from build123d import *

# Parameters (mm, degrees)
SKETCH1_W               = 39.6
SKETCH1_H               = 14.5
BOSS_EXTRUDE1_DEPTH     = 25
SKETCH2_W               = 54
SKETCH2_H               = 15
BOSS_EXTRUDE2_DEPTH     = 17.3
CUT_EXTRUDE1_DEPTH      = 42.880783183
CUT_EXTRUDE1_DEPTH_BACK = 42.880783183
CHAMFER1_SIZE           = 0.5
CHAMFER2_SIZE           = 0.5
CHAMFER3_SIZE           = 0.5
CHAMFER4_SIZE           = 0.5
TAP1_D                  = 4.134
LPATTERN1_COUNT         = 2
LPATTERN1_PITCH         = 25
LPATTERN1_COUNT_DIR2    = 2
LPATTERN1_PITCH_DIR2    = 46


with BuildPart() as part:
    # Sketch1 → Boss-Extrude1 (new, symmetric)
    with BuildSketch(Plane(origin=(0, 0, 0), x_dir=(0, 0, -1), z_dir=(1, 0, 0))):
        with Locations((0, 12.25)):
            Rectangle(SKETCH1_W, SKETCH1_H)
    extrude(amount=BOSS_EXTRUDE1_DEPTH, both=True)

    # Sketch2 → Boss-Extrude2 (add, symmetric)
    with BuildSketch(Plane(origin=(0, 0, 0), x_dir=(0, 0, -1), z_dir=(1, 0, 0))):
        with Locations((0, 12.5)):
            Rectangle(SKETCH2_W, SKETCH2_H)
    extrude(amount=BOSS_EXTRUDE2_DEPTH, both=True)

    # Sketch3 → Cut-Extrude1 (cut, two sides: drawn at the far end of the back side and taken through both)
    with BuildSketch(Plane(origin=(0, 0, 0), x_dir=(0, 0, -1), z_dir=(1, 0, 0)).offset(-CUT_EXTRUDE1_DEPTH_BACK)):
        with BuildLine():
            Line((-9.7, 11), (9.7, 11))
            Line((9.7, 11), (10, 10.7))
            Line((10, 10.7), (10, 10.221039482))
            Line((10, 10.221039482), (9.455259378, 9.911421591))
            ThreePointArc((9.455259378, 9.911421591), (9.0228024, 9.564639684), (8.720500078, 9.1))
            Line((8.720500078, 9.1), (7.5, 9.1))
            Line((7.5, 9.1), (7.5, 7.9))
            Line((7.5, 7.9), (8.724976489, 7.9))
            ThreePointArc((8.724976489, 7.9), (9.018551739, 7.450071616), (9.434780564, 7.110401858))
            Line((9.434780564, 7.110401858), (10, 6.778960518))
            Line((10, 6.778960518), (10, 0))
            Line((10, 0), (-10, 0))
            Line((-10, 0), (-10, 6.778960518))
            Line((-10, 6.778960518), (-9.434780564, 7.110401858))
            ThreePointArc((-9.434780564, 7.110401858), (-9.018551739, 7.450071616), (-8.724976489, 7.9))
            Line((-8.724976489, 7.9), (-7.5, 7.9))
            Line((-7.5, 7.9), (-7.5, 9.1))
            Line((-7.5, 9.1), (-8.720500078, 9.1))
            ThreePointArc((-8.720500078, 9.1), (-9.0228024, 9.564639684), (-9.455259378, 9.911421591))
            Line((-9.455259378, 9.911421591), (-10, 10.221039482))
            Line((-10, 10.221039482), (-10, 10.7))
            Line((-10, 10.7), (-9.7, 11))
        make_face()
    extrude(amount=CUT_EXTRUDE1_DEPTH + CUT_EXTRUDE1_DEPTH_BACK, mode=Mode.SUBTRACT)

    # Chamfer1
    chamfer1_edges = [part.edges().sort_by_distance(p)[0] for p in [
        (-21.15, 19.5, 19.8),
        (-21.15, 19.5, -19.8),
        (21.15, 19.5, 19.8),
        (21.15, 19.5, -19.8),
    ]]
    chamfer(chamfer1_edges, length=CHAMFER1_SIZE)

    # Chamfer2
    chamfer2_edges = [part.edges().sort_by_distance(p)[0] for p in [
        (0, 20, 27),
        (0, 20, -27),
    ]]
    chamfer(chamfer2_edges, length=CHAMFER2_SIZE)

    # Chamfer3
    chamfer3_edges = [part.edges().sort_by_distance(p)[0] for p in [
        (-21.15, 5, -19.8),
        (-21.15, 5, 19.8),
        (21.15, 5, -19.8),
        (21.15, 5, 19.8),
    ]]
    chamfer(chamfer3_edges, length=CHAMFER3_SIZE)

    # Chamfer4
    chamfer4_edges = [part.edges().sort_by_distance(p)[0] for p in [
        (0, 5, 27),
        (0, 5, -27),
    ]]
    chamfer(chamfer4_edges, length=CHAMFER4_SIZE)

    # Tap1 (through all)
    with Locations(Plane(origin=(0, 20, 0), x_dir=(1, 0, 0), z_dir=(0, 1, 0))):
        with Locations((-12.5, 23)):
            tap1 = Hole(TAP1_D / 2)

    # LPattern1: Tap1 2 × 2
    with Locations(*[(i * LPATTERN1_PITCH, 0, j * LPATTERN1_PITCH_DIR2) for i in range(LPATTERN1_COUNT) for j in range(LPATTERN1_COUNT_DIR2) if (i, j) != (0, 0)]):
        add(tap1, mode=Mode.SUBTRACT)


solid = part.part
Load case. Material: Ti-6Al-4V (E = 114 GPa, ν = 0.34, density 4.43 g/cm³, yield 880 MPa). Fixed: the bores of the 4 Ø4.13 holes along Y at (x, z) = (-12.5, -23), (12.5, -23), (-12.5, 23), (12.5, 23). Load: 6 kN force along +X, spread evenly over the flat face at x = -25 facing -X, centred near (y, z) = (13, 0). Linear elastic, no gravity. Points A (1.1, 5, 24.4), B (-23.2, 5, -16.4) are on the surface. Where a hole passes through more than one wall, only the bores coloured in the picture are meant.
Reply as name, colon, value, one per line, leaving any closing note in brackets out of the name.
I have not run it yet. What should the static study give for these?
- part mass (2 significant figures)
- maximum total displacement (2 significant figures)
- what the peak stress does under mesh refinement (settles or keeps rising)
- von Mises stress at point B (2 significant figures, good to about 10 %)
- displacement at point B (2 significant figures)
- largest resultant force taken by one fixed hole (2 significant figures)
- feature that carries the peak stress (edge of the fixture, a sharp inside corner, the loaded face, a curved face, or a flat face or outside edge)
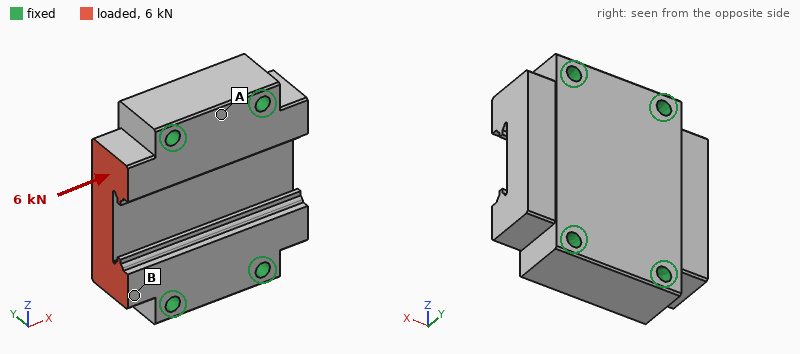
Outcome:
part mass: 140 g
maximum total displacement: 4.0 µm
what the peak stress does under mesh refinement: keeps rising
von Mises stress at point B: 13 MPa
displacement at point B: 2.8 µm
largest resultant force taken by one fixed hole: 1.9 kN
feature that carries the peak stress: edge of the fixture
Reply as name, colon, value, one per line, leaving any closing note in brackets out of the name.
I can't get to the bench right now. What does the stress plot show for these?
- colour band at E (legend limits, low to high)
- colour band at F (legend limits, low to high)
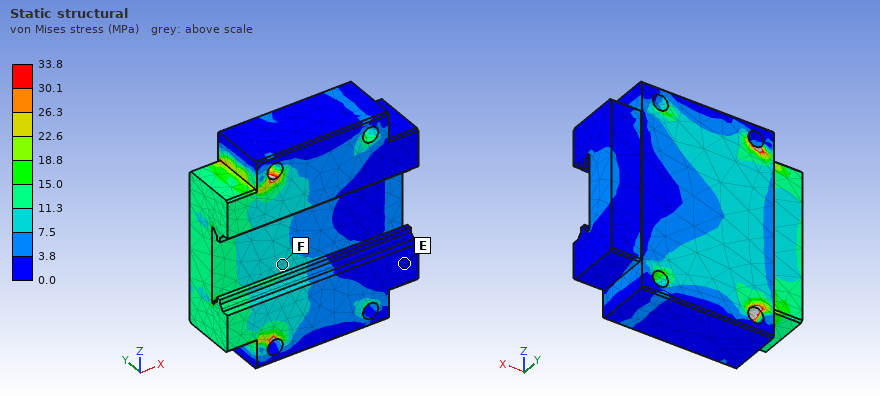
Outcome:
colour band at E: 0.0 to 3.8 MPa
colour band at F: 7.5 to 11.3 MPa
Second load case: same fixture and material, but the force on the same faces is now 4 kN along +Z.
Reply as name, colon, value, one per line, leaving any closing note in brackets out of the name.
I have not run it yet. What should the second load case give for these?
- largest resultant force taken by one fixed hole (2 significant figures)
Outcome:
largest resultant force taken by one fixed hole: 2.1 kN
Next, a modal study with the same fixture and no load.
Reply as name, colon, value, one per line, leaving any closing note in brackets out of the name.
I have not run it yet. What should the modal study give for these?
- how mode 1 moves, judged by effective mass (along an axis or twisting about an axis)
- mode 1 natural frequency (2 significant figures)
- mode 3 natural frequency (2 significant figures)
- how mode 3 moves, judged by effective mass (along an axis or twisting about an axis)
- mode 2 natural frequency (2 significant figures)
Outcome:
how mode 1 moves, judged by effective mass: along Y
mode 1 natural frequency: 20 kHz
mode 3 natural frequency: 30 kHz
how mode 3 moves, judged by effective mass: along X
mode 2 natural frequency: 22 kHz
